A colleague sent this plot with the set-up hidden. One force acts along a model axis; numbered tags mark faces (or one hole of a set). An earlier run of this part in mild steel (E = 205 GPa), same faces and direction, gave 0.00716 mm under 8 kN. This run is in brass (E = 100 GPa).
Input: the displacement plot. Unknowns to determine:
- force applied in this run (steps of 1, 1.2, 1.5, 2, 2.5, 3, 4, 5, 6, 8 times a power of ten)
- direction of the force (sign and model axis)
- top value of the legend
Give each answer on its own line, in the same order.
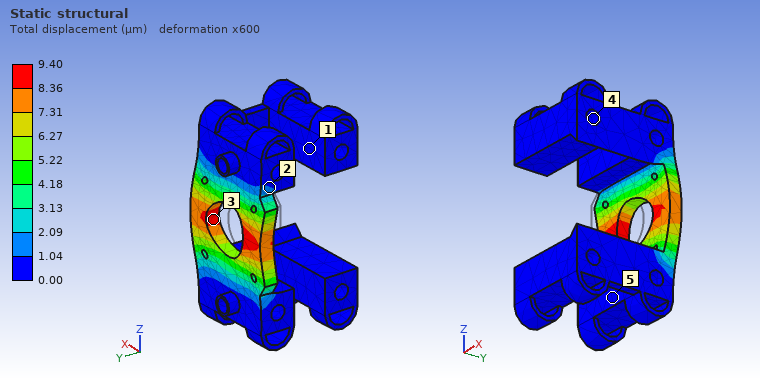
5 kN
+X
9.40 µm
